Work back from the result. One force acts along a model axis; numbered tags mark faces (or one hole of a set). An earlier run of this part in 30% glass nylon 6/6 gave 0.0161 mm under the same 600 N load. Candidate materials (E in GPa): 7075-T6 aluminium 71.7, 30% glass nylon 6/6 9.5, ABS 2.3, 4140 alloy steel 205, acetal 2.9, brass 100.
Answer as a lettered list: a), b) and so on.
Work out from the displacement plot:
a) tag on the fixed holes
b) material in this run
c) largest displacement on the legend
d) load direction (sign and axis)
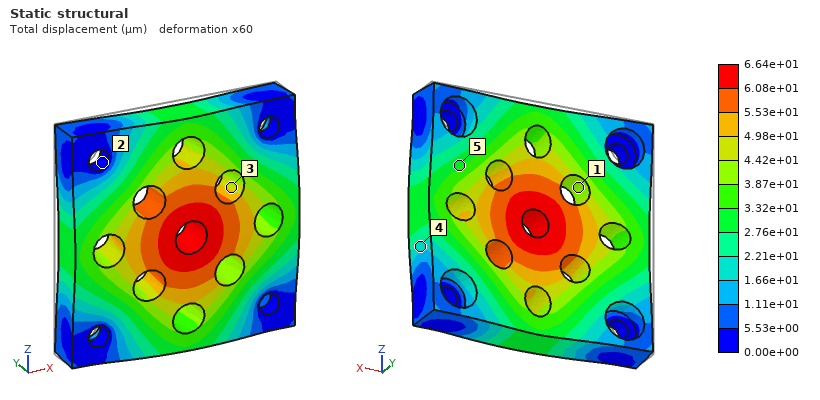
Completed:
a) 2
b) ABS
c) 6.64e+01 µm
d) -Y
